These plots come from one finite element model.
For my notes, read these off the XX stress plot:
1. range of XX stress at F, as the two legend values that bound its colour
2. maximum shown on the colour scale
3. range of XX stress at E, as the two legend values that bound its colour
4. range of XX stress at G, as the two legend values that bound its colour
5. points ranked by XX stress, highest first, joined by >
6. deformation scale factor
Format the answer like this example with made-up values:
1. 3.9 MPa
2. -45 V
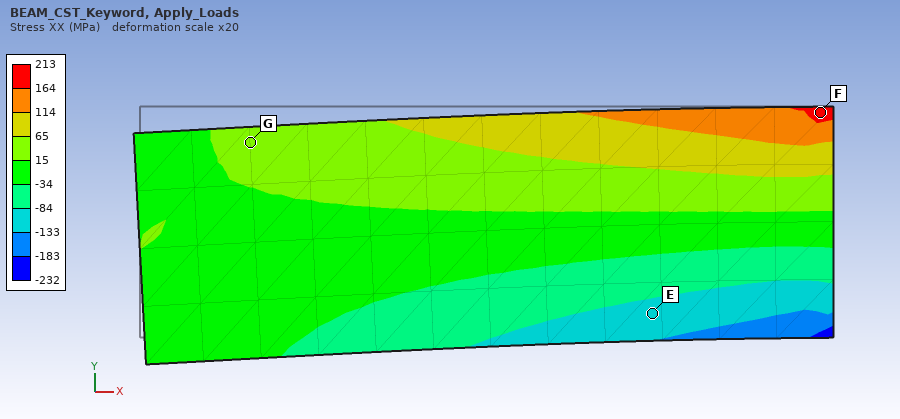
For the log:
1. 164 to 213 MPa
2. 213 MPa
3. -133 to -84 MPa
4. 15 to 65 MPa
5. F > G > E
6. 20
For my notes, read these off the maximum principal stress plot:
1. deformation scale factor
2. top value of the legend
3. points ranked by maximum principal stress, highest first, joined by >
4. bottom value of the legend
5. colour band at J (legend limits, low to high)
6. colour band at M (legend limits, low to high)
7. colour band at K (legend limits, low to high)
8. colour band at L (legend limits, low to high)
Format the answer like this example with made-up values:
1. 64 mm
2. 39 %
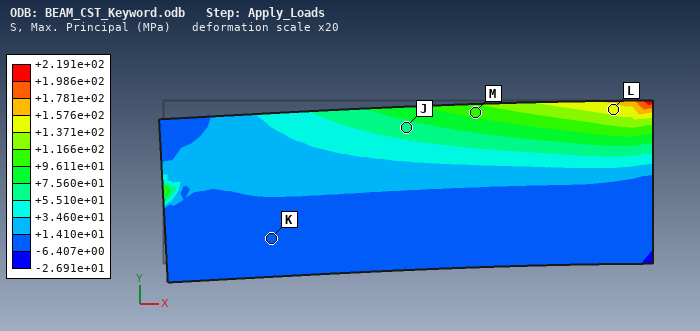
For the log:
1. 20
2. +2.191e+02 MPa
3. L > M > J > K
4. -2.691e+01 MPa
5. +5.510e+01 to +7.560e+01 MPa
6. +9.611e+01 to +1.166e+02 MPa
7. -6.407e+00 to +1.410e+01 MPa
8. +1.371e+02 to +1.576e+02 MPa
